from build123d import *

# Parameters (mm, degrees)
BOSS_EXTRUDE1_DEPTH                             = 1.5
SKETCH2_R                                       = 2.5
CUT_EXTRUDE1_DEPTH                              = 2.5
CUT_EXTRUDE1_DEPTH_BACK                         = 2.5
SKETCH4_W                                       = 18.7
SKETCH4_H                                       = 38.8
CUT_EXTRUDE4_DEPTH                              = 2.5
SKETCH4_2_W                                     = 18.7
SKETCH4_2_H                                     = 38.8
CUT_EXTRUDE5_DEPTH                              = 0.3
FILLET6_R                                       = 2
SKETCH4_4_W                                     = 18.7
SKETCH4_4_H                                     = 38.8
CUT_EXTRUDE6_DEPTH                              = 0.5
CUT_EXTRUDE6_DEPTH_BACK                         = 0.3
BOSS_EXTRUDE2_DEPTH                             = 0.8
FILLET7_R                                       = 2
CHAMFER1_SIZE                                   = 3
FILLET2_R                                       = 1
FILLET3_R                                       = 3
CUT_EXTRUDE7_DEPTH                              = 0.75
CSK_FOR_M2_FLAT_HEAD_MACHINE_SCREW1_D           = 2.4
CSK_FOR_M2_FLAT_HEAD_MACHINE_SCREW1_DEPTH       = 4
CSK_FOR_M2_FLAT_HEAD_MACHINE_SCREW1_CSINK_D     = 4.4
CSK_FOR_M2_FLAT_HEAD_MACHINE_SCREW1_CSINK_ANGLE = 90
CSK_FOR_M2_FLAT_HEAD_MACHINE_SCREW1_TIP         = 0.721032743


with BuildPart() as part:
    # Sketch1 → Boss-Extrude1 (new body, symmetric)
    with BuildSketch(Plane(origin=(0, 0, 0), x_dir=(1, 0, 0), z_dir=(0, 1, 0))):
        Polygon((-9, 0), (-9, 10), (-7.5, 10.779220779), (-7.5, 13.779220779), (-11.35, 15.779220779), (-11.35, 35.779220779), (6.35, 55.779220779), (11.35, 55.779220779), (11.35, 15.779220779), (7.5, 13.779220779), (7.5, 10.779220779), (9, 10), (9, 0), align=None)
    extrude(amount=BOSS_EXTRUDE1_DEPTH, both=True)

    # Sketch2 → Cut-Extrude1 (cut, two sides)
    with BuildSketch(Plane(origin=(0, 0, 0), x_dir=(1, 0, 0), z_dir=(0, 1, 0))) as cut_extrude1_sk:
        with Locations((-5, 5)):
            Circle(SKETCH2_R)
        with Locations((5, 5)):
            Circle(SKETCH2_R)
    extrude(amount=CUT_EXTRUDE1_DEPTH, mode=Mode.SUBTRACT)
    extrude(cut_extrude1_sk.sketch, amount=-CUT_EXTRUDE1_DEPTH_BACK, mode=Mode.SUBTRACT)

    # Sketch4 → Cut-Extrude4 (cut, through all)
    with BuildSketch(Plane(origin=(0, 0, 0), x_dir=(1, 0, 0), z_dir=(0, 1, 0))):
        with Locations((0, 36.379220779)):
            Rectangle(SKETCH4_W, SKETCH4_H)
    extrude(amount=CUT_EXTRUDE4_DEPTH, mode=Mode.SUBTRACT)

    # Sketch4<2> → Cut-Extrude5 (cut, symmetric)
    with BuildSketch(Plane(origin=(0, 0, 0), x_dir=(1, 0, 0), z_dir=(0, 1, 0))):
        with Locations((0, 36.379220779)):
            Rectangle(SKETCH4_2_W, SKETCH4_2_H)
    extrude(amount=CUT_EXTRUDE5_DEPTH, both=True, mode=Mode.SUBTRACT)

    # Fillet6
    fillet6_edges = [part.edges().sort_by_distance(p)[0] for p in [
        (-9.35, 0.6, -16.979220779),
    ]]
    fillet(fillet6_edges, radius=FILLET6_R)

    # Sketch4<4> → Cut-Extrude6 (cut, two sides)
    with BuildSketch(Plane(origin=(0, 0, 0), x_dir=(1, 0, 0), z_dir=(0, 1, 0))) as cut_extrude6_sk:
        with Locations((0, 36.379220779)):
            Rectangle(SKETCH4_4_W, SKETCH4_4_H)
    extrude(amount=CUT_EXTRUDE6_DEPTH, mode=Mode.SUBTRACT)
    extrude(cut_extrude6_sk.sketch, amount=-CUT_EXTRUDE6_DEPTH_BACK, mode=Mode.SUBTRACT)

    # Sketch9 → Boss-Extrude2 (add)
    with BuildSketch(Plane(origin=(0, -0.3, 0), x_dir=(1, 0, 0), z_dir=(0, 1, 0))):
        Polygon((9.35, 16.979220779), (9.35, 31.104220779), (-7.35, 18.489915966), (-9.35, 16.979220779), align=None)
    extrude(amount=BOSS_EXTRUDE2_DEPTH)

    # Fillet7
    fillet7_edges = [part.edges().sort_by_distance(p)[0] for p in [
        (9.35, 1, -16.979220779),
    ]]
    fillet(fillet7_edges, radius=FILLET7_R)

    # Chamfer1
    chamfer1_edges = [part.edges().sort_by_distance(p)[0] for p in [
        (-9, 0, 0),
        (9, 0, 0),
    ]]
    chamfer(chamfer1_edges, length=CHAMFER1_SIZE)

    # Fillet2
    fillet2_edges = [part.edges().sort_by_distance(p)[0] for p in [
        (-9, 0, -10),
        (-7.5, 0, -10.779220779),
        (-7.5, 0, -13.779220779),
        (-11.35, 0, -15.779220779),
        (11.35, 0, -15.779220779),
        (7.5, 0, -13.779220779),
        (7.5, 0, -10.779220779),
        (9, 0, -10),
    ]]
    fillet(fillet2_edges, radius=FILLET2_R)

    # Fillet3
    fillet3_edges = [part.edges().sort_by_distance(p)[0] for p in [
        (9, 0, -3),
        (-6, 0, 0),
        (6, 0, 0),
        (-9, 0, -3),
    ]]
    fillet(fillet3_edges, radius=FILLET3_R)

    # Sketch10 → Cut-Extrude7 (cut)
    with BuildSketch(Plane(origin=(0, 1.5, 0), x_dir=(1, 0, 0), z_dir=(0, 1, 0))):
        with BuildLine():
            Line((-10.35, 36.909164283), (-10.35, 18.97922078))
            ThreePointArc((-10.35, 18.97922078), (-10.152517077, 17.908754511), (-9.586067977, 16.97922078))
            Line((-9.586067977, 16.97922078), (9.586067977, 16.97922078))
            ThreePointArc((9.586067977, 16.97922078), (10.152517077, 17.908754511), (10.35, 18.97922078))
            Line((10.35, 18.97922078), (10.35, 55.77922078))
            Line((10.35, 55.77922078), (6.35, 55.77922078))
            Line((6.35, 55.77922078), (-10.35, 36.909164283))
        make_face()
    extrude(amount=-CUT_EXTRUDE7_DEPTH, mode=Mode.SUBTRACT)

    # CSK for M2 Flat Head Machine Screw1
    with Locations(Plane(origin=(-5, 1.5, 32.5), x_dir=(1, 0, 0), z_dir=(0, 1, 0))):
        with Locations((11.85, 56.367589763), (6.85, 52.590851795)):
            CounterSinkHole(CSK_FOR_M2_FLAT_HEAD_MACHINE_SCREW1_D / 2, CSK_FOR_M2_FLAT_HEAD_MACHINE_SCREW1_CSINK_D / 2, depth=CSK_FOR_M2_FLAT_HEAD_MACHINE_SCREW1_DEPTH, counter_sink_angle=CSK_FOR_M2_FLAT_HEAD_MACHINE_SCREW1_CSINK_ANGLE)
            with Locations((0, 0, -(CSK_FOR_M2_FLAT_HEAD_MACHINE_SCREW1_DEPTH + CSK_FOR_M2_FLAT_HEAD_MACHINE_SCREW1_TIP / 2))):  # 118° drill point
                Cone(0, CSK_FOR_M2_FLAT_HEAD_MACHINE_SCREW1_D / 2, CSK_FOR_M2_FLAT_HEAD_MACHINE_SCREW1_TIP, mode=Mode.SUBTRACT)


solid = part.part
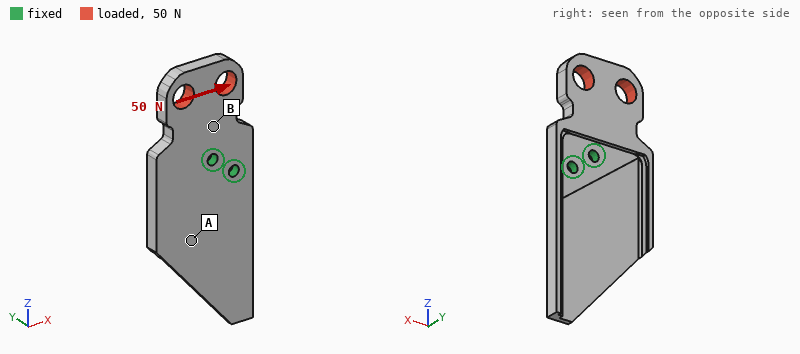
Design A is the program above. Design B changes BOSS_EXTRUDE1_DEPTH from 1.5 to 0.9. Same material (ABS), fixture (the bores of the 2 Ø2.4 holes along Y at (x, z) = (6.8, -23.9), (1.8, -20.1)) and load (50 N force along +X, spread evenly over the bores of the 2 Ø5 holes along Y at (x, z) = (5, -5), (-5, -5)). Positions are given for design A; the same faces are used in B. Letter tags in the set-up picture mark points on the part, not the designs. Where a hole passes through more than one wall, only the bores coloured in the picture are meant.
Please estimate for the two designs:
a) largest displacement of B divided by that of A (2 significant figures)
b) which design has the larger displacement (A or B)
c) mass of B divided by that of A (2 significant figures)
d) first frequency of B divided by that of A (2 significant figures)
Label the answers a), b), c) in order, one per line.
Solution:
a) 1.6
b) B
c) 0.59
d) 0.67
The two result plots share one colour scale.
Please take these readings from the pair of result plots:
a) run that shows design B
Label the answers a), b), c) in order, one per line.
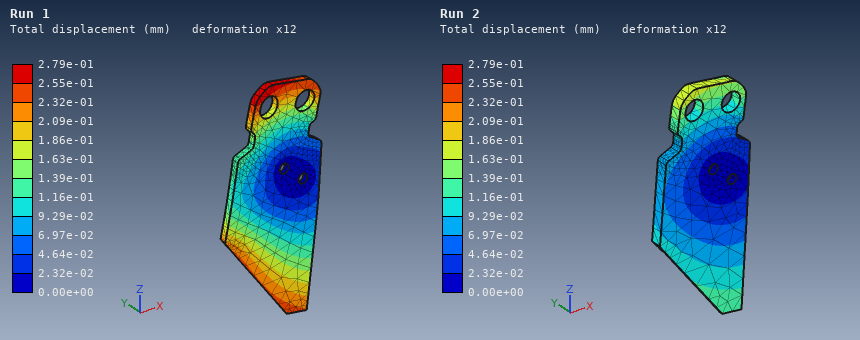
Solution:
a) Run 1
